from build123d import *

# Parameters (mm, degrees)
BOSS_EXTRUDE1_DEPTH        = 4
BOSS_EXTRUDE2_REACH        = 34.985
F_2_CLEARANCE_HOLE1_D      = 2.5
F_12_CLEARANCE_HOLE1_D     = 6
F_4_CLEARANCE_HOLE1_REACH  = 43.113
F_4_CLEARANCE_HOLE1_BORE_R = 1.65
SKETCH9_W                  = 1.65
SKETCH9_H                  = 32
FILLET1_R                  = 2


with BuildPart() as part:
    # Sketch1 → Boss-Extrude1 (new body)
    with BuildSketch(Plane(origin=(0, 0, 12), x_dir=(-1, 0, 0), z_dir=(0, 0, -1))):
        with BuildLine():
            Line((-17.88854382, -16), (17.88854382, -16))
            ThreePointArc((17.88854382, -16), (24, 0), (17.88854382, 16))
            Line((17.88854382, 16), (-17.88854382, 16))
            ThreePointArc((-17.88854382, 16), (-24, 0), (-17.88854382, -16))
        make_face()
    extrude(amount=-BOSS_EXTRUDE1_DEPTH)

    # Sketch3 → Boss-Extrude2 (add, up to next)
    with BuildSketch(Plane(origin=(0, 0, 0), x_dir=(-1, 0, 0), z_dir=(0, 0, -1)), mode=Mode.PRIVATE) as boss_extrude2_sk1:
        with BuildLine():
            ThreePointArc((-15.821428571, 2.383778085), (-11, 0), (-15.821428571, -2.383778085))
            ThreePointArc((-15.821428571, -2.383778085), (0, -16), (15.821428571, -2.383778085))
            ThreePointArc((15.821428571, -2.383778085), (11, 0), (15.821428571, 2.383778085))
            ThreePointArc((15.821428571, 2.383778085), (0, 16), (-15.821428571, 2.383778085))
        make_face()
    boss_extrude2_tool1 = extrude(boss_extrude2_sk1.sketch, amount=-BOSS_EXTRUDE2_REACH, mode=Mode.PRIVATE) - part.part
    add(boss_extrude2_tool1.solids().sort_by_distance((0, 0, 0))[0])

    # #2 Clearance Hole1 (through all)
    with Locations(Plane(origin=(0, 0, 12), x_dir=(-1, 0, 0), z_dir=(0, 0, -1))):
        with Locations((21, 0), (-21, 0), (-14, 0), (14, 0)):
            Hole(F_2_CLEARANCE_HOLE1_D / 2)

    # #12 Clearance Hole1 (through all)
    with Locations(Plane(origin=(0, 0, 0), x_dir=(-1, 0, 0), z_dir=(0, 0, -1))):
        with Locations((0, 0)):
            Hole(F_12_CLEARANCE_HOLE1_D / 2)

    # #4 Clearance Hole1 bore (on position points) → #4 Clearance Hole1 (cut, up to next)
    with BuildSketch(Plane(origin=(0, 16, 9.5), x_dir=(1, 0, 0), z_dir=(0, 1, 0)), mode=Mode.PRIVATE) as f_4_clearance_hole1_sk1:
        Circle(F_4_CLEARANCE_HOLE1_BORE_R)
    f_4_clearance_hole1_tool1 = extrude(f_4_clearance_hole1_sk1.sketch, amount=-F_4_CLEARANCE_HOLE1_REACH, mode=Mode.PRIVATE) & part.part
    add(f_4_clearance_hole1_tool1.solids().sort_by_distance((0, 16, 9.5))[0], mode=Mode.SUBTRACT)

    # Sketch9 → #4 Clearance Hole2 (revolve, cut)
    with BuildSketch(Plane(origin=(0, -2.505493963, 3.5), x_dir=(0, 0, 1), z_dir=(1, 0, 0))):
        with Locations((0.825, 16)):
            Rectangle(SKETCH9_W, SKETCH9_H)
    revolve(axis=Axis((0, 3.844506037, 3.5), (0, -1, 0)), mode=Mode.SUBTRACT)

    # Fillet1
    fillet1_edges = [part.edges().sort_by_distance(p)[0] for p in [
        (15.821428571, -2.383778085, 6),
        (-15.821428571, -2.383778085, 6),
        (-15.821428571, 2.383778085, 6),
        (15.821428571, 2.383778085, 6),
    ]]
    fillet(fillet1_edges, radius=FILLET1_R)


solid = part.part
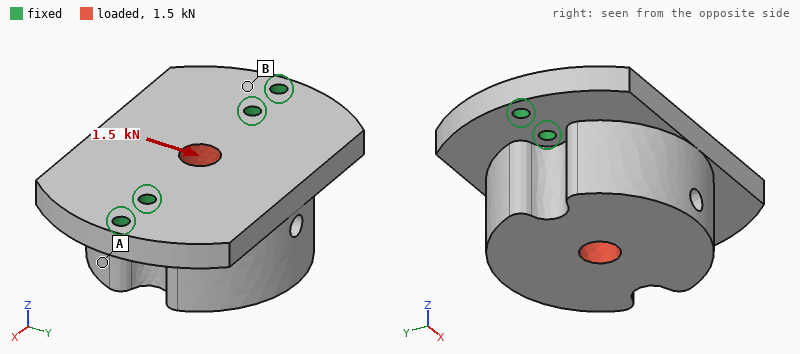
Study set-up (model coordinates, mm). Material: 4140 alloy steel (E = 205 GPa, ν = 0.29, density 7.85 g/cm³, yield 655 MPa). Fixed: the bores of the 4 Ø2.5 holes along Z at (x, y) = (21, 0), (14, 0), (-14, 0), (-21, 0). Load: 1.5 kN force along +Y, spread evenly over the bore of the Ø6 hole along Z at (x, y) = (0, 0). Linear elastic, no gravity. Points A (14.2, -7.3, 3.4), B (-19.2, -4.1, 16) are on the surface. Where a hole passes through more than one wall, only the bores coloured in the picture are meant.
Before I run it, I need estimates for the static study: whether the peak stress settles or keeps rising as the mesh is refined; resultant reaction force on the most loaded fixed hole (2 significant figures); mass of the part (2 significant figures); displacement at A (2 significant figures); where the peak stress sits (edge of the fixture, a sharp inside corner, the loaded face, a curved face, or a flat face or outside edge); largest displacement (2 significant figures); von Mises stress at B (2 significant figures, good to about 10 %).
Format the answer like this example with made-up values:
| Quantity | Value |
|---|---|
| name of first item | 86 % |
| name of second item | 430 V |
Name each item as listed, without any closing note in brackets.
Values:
| Quantity | Value |
|---|---|
| whether the peak stress settles or keeps rising as the mesh is refined | keeps rising |
| resultant reaction force on the most loaded fixed hole | 710 N |
| mass of the part | 110 g |
| displacement at A | 7.3 µm |
| where the peak stress sits | edge of the fixture |
| largest displacement | 12 µm |
| von Mises stress at B | 25 MPa |
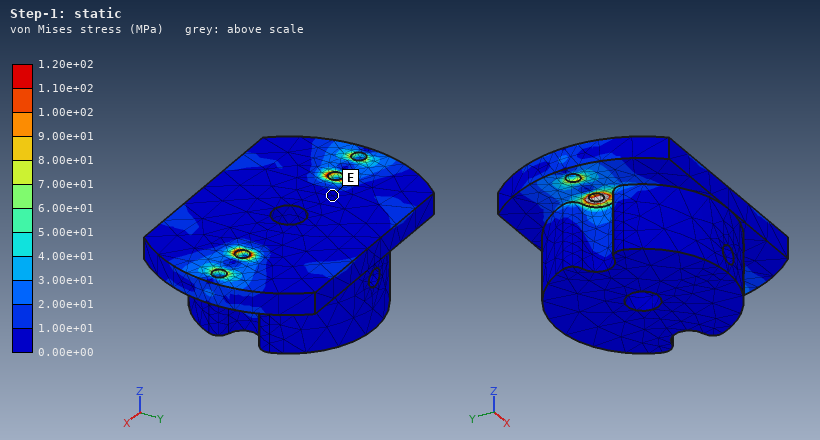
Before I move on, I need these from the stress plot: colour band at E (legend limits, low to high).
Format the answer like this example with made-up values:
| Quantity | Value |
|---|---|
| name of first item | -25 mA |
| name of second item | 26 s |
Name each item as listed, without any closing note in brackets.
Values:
| Quantity | Value |
|---|---|
| colour band at E | 0.00e+00 to 1.00e+01 MPa |
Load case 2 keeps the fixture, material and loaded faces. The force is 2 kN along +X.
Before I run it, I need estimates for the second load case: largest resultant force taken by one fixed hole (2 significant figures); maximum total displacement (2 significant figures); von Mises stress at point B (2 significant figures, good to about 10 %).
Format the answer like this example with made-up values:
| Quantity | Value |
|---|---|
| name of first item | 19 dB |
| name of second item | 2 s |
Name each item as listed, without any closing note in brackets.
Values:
| Quantity | Value |
|---|---|
| largest resultant force taken by one fixed hole | 840 N |
| maximum total displacement | 1.5 µm |
| von Mises stress at point B | 8.8 MPa |
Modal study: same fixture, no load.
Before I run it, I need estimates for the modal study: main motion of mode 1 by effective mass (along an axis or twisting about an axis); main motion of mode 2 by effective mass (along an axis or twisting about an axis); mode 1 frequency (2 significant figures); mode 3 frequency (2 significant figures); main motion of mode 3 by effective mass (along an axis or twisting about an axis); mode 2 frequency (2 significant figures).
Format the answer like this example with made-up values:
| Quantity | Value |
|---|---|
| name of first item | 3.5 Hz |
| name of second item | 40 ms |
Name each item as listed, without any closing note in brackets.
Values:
| Quantity | Value |
|---|---|
| main motion of mode 1 by effective mass | along Y |
| main motion of mode 2 by effective mass | along Z |
| mode 1 frequency | 5700 Hz |
| mode 3 frequency | 21 kHz |
| main motion of mode 3 by effective mass | along X |
| mode 2 frequency | 17 kHz |
